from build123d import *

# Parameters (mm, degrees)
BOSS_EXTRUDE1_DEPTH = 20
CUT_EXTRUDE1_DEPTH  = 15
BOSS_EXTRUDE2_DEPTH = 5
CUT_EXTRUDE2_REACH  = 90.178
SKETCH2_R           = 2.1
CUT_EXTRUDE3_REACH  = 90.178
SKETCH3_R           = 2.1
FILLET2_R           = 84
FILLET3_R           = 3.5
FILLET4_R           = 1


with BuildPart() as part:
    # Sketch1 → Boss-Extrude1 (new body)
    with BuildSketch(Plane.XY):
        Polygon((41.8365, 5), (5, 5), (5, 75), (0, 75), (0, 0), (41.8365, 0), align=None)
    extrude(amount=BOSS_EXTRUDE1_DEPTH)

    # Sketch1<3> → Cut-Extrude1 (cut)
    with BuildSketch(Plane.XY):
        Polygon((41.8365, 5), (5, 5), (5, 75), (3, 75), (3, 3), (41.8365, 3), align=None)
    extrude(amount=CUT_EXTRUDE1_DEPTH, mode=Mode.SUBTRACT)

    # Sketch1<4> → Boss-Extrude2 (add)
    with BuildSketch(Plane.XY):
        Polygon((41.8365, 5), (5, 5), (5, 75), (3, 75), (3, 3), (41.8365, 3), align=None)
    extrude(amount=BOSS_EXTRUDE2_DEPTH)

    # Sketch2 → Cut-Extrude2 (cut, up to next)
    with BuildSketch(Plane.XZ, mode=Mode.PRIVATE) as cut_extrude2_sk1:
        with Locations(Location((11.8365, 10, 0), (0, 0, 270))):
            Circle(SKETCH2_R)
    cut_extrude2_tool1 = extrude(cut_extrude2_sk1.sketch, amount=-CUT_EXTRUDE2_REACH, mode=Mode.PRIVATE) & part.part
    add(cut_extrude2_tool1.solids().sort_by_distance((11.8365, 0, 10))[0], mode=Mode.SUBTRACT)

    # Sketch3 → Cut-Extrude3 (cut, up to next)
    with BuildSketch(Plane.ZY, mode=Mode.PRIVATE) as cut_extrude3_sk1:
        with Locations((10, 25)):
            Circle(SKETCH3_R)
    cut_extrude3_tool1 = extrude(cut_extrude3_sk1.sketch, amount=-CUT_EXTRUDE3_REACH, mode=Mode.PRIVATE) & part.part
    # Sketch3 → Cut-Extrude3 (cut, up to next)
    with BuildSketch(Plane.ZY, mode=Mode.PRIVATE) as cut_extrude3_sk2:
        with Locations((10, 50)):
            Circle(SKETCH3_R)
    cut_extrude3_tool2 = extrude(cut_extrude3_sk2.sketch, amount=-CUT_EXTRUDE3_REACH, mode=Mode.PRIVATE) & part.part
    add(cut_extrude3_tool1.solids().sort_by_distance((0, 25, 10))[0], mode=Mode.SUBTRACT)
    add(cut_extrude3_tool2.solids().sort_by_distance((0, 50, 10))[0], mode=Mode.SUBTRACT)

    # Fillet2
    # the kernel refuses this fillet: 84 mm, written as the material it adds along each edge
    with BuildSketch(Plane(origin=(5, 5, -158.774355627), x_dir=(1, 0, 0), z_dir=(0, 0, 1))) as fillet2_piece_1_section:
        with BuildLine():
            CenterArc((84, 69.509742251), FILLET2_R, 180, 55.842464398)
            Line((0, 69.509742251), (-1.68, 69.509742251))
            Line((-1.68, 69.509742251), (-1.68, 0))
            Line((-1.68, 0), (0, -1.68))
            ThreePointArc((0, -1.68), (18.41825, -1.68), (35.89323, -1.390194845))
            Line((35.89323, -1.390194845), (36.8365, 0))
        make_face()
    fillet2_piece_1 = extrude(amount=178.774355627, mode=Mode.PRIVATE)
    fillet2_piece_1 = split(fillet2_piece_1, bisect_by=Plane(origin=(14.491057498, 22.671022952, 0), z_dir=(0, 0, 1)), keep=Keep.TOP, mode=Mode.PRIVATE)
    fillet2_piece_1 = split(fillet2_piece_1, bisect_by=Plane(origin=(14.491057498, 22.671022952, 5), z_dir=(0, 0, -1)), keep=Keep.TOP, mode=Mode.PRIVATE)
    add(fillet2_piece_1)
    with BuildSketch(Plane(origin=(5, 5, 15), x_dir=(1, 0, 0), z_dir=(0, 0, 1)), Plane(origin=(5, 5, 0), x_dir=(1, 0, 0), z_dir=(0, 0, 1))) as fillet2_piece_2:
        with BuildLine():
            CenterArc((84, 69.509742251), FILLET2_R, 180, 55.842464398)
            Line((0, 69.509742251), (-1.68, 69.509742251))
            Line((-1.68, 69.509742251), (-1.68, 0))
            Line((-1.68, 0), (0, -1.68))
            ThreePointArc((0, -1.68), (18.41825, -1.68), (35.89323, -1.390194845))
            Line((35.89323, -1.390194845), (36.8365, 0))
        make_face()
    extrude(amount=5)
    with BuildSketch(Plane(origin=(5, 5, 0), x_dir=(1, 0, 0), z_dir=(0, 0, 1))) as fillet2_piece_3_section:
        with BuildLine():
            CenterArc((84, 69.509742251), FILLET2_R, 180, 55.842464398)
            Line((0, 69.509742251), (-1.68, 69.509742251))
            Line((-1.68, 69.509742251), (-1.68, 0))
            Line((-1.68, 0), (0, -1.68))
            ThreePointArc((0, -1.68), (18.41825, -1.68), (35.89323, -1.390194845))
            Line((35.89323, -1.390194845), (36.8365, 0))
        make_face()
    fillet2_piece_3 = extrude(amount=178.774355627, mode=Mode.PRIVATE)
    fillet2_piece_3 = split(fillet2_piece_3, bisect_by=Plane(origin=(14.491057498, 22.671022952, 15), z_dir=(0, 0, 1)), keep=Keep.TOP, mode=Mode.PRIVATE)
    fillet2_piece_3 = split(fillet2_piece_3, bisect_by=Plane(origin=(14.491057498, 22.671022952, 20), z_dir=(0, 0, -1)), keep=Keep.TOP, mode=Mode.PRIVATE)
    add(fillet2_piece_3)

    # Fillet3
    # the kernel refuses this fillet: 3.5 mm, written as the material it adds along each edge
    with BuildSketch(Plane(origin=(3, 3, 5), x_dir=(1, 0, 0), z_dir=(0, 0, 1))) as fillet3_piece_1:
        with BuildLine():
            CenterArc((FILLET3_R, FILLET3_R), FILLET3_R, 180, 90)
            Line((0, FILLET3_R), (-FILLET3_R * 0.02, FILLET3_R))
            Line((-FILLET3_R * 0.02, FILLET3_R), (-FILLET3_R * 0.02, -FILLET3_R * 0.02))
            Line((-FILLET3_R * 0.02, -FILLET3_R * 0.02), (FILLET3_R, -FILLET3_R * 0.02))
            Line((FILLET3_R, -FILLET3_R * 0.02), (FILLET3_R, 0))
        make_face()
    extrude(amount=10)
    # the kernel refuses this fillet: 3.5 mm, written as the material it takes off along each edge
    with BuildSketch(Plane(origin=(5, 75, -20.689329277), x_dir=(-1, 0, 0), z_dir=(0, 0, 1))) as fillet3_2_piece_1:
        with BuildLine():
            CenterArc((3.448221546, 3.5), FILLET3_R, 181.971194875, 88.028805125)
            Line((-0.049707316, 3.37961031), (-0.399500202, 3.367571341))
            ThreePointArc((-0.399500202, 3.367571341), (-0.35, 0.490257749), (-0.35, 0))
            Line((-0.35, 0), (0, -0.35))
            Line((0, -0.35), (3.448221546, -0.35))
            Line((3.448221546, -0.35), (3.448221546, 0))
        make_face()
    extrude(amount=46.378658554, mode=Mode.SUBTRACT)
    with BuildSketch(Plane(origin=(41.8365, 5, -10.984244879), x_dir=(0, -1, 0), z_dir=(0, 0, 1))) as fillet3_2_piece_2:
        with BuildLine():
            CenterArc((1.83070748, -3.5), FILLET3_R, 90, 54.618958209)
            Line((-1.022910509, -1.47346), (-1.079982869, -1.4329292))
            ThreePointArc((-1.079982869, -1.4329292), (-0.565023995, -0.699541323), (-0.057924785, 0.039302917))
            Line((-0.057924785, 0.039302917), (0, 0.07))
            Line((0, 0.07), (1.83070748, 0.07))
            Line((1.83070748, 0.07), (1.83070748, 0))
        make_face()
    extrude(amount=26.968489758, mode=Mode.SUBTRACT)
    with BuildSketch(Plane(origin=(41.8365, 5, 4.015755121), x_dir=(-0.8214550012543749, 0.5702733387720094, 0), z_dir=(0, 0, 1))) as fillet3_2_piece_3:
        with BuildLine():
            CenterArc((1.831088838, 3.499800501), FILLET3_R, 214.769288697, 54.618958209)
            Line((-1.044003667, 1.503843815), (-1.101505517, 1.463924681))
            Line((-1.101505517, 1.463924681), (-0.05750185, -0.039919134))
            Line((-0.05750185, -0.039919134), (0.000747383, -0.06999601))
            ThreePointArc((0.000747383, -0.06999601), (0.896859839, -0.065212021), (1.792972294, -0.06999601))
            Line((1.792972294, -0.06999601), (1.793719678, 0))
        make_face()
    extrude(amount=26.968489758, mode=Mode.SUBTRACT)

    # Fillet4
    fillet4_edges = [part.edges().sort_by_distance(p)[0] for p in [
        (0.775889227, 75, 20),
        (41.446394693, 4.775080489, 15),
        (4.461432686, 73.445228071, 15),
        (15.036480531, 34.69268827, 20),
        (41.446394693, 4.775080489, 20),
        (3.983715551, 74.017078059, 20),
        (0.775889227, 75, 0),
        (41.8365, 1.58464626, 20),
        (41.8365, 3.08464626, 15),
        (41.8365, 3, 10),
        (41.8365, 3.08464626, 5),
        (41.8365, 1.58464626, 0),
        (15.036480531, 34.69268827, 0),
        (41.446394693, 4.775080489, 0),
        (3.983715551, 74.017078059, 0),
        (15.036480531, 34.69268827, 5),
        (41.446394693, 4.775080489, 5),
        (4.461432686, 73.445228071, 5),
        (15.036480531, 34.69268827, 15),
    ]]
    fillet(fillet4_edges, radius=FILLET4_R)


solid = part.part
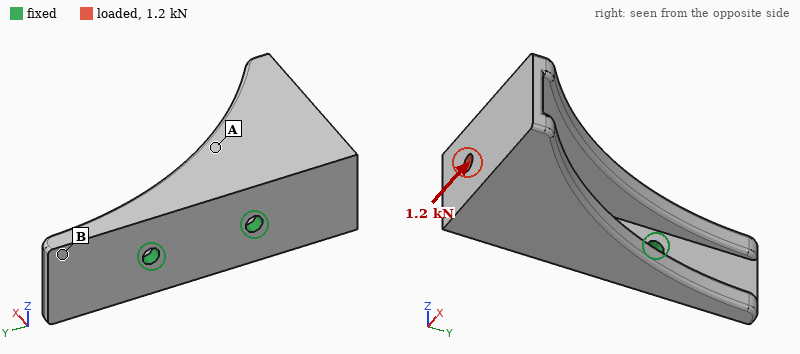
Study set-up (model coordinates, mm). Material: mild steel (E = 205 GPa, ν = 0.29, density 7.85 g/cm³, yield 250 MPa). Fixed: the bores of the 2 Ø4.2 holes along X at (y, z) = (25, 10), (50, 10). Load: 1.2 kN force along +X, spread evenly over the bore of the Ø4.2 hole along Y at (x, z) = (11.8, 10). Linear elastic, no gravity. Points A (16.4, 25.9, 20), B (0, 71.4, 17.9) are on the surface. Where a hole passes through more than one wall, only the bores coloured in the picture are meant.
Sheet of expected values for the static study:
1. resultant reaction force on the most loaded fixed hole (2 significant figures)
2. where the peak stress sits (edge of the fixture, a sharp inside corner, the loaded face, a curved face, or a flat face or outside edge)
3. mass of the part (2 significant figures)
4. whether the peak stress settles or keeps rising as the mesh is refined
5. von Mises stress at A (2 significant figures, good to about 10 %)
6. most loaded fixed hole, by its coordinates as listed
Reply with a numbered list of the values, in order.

1. 2.3 kN
2. edge of the fixture
3. 130 g
4. keeps rising
5. 32 MPa
6. (25, 10)
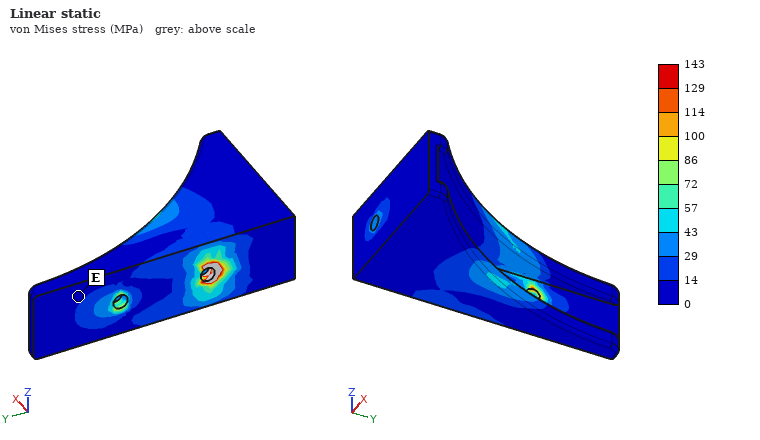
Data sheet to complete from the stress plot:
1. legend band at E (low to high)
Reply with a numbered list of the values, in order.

1. 0 to 14 MPa
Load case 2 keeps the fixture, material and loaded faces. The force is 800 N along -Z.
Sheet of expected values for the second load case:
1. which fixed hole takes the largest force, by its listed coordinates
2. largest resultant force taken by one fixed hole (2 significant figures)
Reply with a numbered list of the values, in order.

1. (25, 10)
2. 1.4 kN
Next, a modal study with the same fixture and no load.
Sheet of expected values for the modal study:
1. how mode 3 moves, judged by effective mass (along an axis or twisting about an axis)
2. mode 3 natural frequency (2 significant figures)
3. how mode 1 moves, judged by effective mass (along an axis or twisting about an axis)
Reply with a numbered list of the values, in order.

1. along X
2. 8000 Hz
3. along Z
